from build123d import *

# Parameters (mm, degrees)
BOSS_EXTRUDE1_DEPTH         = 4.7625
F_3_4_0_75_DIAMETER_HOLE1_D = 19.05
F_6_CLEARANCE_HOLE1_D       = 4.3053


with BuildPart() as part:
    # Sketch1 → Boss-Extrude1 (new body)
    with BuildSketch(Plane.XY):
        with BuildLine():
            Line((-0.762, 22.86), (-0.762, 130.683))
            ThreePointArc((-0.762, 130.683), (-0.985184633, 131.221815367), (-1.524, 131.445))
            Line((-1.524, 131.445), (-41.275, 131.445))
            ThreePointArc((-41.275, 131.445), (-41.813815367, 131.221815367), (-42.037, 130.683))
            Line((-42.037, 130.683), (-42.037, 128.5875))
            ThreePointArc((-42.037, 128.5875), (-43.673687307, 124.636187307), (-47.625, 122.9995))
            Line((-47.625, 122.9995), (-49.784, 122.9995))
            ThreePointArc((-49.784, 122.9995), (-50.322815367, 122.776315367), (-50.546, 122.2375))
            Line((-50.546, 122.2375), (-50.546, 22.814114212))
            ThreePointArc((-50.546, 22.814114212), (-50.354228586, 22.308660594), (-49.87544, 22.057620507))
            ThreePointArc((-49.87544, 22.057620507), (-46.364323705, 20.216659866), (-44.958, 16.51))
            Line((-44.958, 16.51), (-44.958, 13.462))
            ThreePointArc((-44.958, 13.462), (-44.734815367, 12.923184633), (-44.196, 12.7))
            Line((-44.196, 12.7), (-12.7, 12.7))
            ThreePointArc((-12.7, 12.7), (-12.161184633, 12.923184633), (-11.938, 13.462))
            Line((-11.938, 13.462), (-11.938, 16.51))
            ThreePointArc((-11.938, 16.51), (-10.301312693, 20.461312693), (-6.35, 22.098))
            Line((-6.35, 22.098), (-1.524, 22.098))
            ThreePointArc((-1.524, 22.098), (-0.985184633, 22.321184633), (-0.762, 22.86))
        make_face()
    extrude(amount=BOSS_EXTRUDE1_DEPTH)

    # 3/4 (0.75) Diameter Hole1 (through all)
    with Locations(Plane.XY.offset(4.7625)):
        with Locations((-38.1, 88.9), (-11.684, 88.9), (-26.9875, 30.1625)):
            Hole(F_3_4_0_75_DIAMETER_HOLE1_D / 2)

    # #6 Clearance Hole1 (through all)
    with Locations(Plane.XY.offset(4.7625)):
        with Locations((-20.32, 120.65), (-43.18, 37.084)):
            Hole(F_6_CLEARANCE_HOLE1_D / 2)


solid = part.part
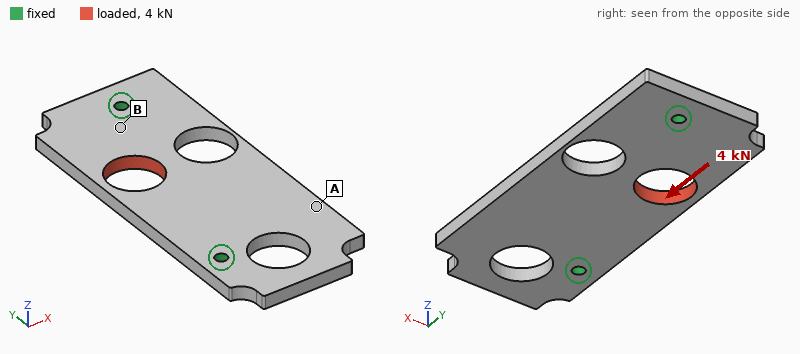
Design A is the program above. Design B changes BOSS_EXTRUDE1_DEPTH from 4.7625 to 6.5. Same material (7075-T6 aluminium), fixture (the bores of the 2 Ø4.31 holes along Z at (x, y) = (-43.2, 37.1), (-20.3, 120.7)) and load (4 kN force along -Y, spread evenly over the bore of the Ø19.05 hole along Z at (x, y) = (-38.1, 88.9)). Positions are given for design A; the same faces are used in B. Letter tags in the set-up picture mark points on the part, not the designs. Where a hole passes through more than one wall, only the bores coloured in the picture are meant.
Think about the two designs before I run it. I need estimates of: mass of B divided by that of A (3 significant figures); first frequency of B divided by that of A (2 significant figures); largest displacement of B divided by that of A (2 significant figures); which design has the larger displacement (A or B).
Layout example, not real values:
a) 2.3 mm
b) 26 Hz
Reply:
a) 1.36
b) 1.3
c) 0.72
d) A
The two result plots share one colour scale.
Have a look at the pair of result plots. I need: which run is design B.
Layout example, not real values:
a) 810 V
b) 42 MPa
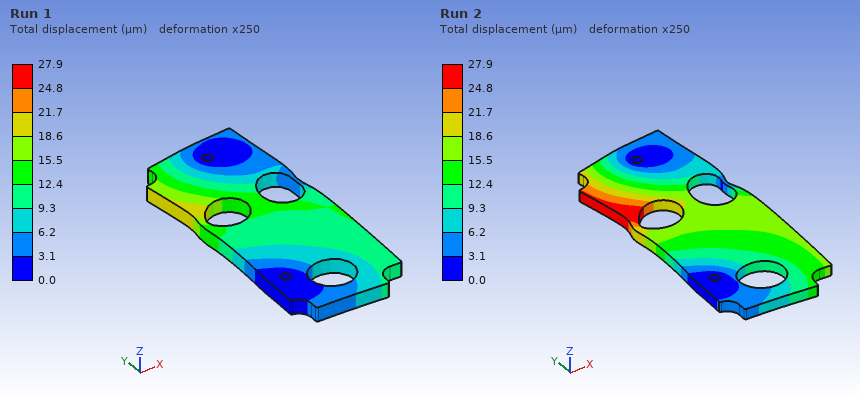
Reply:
a) Run 1
